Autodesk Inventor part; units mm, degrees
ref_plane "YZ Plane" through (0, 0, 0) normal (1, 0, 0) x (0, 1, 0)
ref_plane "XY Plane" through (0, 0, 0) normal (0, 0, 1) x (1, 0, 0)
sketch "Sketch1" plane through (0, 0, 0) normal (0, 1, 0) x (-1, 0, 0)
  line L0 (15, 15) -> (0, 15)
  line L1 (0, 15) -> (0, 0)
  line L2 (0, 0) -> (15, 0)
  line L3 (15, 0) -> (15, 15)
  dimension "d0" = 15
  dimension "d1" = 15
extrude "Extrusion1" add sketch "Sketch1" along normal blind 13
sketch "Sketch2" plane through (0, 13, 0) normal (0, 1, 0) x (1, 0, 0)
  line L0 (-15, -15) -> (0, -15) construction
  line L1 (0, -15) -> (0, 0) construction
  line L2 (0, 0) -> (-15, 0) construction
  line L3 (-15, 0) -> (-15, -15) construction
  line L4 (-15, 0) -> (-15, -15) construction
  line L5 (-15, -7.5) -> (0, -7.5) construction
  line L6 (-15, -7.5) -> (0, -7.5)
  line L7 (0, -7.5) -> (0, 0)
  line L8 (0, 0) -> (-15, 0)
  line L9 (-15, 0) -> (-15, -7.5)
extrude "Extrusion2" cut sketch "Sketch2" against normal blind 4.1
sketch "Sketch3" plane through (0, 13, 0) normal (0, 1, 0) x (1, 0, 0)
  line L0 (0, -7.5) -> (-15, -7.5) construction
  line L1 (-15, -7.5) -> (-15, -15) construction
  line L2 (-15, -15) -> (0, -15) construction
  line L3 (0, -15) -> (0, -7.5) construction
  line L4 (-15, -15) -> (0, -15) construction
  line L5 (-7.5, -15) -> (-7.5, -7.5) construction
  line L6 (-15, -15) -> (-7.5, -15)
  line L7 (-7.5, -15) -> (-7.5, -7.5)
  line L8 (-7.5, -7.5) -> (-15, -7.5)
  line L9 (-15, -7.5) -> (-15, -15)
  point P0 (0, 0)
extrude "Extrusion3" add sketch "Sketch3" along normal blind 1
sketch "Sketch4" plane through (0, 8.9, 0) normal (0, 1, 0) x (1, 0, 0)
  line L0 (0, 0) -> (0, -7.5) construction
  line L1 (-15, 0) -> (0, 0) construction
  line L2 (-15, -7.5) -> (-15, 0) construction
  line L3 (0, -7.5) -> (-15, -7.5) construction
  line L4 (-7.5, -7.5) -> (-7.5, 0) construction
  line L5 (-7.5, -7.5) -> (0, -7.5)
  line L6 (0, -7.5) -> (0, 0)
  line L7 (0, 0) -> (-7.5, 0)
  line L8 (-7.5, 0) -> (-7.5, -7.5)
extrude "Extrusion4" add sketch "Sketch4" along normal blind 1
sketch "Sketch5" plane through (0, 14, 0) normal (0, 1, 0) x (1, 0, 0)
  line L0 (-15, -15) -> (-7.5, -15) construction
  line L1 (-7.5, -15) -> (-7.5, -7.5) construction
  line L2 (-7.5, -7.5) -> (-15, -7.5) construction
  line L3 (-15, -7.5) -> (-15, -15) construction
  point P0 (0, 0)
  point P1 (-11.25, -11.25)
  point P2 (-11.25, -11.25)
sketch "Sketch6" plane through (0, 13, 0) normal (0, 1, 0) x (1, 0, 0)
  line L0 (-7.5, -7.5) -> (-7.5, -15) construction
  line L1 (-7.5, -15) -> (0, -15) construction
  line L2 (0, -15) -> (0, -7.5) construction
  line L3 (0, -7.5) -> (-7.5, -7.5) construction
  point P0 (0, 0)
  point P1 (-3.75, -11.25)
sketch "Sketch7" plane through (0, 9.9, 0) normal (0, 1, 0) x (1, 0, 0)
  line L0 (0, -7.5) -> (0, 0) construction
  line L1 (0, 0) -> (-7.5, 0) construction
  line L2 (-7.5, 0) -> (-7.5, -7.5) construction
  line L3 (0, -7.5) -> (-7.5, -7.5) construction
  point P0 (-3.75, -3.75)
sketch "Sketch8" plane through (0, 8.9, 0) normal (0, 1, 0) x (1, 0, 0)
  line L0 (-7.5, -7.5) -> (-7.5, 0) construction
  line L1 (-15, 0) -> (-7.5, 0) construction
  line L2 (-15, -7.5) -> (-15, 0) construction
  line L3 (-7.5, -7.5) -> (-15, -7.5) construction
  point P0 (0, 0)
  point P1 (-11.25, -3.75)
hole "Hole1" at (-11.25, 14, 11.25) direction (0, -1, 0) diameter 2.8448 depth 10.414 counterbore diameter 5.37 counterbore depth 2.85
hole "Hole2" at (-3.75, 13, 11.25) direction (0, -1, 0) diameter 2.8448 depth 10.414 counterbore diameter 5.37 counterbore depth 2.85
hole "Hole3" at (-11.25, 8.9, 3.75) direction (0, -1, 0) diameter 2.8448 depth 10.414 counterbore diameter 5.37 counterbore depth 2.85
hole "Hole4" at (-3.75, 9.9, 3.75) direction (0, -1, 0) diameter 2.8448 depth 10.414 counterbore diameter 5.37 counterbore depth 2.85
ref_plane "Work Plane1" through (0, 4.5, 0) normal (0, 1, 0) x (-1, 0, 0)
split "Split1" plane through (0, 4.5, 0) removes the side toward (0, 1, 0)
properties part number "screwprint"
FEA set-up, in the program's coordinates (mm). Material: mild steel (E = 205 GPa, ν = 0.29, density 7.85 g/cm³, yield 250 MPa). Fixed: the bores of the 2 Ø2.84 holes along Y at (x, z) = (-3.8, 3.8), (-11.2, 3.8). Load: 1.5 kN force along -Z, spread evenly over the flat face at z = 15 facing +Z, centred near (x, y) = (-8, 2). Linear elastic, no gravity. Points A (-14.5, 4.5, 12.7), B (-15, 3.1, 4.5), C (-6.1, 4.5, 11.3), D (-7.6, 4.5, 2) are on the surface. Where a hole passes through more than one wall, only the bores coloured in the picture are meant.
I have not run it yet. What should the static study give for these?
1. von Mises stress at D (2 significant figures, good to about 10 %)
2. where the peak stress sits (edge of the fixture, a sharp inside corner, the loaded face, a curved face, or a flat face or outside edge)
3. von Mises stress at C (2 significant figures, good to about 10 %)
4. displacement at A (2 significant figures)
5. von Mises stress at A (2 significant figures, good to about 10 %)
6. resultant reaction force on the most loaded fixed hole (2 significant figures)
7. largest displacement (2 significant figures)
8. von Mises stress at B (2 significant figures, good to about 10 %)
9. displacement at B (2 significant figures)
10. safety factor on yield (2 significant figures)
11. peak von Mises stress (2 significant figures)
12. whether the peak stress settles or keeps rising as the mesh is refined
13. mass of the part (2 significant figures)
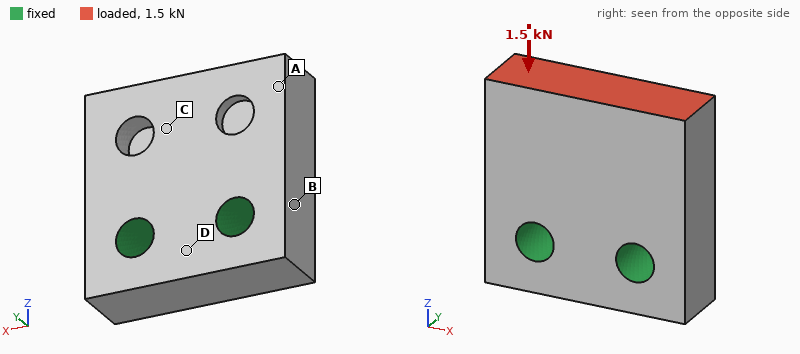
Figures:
4.5 MPa
a curved face
29 MPa
1.1 µm
25 MPa
760 N
1.7 µm
12 MPa
0.31 µm
3.7
68 MPa
settles
7.4 g
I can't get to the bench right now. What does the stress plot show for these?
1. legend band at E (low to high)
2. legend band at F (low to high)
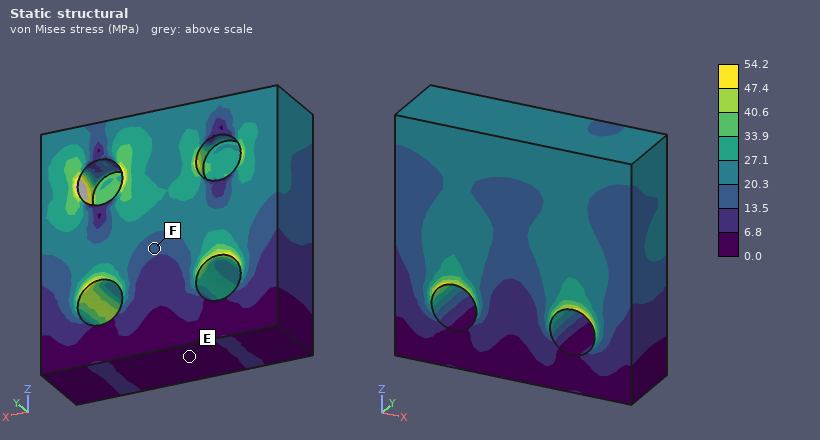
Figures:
0.0 to 6.8 MPa
13.5 to 20.3 MPa
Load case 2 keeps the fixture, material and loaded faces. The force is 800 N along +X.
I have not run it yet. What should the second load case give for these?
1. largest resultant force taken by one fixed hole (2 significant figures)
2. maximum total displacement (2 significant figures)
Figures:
970 N
4.6 µm
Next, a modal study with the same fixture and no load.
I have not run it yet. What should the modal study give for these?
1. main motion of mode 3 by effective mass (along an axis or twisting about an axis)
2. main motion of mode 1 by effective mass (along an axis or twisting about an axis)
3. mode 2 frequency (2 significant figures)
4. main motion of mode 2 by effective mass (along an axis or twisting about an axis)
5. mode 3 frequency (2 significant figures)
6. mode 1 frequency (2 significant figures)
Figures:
along X
along Y
46 kHz
twisting about Z
52 kHz
29 kHz
